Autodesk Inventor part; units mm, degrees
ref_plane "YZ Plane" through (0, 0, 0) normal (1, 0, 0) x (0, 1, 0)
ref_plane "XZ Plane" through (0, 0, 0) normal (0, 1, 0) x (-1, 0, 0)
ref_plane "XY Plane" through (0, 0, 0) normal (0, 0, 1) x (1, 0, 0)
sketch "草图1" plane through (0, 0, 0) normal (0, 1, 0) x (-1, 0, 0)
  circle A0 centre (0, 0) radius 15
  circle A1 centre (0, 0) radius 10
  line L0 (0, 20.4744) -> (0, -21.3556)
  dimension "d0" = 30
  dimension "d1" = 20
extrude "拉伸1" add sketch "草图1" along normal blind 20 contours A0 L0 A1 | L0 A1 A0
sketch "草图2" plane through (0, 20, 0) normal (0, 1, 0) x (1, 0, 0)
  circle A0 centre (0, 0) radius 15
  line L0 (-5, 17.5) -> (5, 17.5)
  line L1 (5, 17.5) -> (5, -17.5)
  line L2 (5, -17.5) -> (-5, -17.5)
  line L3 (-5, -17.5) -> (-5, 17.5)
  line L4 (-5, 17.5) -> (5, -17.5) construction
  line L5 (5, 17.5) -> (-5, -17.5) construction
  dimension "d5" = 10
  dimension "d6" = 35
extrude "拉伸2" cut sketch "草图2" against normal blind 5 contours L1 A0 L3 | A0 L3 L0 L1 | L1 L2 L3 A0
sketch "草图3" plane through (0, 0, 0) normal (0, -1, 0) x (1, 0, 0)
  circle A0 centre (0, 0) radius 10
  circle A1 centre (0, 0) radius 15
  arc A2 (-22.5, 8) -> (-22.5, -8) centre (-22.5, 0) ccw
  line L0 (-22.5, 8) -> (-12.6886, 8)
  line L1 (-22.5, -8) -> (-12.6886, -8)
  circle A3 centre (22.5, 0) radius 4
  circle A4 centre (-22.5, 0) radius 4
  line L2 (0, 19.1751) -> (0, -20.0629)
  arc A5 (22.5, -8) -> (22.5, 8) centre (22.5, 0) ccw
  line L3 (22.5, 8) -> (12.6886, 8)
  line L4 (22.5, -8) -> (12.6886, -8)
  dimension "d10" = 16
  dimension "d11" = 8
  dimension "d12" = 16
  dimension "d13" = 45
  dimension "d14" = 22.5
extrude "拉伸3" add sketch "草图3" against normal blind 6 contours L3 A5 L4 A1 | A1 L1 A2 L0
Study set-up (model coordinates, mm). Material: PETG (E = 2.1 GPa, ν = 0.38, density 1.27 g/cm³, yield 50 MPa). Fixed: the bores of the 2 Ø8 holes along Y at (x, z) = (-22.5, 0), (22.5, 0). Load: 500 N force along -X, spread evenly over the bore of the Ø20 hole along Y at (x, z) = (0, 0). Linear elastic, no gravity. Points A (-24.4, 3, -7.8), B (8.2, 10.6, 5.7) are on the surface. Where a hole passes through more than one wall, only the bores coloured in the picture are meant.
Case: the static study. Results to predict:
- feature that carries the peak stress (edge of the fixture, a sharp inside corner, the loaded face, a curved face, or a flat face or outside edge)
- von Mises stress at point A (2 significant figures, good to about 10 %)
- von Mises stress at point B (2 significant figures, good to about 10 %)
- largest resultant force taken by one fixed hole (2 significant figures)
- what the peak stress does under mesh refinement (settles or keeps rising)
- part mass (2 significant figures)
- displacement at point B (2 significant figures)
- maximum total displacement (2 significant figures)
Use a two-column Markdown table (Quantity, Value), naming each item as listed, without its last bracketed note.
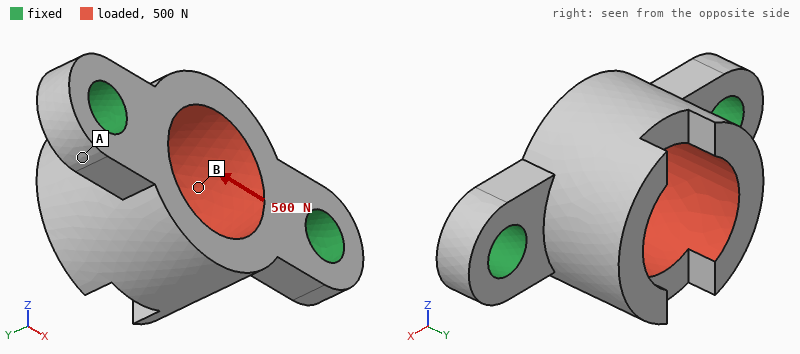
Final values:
| Quantity | Value |
|---|---|
| feature that carries the peak stress | edge of the fixture |
| von Mises stress at point A | 0.70 MPa |
| von Mises stress at point B | 2.2 MPa |
| largest resultant force taken by one fixed hole | 270 N |
| what the peak stress does under mesh refinement | keeps rising |
| part mass | 12 g |
| displacement at point B | 30 µm |
| maximum total displacement | 55 µm |
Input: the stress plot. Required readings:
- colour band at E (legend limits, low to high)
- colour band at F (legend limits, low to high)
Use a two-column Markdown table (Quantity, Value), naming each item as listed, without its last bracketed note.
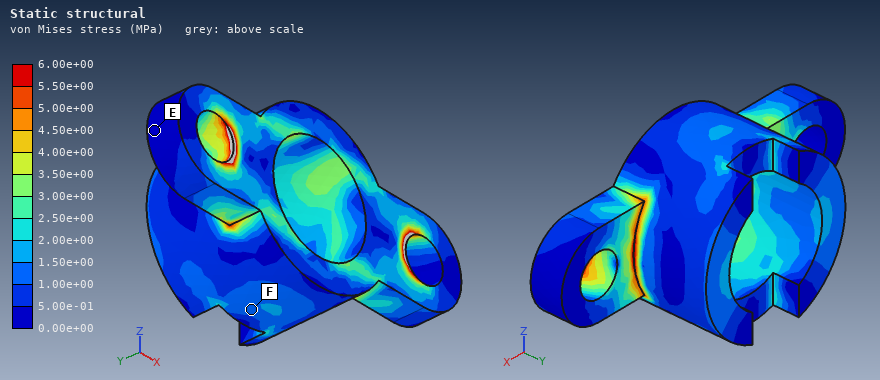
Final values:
| Quantity | Value |
|---|---|
| colour band at E | 0.00e+00 to 5.00e-01 MPa |
| colour band at F | 1.00e+00 to 1.50e+00 MPa |
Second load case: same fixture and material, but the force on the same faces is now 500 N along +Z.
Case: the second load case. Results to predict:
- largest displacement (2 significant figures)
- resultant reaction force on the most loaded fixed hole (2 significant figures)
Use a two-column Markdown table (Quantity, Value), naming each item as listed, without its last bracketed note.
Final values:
| Quantity | Value |
|---|---|
| largest displacement | 0.35 mm |
| resultant reaction force on the most loaded fixed hole | 250 N |
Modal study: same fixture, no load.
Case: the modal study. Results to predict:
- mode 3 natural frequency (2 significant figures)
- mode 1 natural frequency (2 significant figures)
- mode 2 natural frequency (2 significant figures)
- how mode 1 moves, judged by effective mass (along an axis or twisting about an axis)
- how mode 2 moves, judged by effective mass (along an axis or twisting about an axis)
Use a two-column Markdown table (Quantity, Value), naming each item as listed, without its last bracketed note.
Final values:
| Quantity | Value |
|---|---|
| mode 3 natural frequency | 5000 Hz |
| mode 1 natural frequency | 2000 Hz |
| mode 2 natural frequency | 3600 Hz |
| how mode 1 moves, judged by effective mass | along Z |
| how mode 2 moves, judged by effective mass | along Y |
